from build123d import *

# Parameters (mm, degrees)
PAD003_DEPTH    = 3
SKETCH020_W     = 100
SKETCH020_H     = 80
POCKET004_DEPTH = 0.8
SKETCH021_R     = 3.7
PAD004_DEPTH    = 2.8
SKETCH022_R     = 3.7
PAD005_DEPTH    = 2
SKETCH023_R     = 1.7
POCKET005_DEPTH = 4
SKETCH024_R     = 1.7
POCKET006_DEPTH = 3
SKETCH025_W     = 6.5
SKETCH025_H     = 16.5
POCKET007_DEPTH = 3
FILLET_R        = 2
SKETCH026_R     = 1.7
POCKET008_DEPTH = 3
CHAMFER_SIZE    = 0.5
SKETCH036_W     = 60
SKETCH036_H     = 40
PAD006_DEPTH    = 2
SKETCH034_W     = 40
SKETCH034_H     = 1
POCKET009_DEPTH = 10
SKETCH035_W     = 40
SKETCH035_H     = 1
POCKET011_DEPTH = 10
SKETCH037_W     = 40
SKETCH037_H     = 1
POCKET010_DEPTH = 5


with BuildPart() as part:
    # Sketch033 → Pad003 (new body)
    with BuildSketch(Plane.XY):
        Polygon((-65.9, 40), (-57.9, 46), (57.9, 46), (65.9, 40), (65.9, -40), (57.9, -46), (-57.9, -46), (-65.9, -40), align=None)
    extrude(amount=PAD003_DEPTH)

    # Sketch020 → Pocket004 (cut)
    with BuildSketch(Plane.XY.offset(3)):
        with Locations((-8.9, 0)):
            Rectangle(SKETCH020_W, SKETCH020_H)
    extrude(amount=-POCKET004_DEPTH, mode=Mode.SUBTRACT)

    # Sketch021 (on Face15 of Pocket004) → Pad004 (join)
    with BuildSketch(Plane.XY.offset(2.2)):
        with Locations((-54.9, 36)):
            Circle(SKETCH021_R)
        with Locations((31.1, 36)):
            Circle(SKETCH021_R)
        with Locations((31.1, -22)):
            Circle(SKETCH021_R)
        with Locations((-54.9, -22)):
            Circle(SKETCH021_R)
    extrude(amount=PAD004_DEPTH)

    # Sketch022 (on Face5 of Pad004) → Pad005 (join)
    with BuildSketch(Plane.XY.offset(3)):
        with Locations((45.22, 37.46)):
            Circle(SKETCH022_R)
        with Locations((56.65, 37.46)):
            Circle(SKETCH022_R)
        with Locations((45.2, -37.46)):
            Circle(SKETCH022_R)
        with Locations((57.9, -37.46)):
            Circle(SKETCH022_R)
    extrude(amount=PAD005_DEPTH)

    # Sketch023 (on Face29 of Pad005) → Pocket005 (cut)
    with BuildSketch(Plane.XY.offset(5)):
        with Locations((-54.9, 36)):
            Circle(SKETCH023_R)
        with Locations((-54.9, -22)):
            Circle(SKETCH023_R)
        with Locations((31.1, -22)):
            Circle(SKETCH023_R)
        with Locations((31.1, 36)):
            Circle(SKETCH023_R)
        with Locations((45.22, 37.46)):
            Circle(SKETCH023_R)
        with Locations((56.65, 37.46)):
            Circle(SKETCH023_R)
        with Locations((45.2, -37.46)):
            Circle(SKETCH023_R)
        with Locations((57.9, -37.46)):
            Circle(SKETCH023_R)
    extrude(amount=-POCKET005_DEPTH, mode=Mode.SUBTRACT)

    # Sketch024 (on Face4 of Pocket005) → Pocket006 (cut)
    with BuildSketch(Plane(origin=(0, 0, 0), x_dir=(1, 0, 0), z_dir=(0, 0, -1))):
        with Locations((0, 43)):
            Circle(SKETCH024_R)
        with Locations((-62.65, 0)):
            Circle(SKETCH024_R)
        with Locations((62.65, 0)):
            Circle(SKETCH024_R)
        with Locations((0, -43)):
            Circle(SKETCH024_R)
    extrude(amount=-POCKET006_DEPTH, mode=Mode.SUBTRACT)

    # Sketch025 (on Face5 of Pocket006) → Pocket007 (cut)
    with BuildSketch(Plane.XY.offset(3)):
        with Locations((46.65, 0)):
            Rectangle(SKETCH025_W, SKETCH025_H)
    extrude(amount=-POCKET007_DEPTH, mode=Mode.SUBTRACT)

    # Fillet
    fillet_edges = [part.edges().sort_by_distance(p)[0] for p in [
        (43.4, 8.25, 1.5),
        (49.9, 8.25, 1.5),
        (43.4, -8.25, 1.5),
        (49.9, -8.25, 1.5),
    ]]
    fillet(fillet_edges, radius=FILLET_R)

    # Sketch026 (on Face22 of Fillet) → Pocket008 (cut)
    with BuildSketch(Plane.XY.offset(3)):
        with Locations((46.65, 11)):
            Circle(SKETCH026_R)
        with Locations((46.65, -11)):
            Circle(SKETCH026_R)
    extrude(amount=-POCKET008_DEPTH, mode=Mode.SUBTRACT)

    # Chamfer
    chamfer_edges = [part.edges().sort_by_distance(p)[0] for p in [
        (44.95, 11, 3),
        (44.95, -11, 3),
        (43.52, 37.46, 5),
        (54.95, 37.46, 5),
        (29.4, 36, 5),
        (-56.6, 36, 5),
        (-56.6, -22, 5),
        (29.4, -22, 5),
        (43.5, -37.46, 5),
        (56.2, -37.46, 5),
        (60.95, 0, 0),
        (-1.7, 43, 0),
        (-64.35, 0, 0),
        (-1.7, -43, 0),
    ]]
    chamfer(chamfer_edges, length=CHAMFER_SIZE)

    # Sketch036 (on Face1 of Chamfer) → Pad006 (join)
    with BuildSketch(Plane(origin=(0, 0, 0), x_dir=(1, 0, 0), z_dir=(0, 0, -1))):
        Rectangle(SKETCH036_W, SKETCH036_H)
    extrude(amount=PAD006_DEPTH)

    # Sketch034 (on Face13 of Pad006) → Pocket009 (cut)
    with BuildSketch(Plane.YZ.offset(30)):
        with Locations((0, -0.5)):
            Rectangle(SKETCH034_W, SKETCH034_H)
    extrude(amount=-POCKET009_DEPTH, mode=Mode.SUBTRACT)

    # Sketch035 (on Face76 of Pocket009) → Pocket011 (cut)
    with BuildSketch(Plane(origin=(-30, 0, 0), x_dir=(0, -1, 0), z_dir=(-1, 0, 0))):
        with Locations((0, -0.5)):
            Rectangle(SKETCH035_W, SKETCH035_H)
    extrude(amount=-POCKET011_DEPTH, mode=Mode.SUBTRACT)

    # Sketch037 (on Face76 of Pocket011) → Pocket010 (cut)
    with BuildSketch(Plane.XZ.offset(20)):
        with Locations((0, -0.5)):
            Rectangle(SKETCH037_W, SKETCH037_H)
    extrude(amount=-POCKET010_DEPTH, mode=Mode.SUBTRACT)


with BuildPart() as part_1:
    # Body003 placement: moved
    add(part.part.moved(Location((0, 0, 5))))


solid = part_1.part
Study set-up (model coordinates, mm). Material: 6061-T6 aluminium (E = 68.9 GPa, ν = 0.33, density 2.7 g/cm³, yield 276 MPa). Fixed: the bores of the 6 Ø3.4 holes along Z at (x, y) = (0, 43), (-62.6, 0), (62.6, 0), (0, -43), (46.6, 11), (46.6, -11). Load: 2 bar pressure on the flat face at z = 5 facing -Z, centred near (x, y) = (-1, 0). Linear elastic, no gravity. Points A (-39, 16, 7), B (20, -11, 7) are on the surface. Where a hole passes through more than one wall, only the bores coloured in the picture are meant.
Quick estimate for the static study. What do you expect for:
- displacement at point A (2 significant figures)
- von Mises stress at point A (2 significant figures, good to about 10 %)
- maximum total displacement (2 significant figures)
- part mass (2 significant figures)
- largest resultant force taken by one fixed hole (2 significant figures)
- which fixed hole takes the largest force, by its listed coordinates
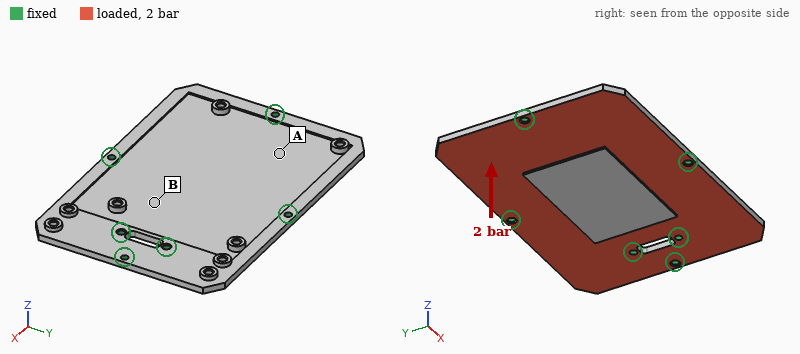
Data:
0.23 mm
51 MPa
0.57 mm
91 g
640 N
(-62.6, 0)
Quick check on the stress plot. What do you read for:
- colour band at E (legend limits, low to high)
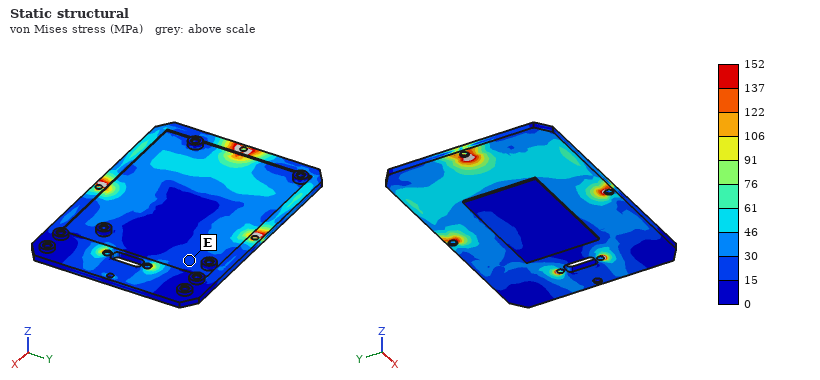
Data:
15 to 30 MPa
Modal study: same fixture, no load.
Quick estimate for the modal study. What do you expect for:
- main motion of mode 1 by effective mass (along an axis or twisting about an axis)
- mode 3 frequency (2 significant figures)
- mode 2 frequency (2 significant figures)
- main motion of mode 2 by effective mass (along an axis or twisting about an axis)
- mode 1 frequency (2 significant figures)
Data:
twisting about X
1900 Hz
1500 Hz
along Z
1400 Hz
